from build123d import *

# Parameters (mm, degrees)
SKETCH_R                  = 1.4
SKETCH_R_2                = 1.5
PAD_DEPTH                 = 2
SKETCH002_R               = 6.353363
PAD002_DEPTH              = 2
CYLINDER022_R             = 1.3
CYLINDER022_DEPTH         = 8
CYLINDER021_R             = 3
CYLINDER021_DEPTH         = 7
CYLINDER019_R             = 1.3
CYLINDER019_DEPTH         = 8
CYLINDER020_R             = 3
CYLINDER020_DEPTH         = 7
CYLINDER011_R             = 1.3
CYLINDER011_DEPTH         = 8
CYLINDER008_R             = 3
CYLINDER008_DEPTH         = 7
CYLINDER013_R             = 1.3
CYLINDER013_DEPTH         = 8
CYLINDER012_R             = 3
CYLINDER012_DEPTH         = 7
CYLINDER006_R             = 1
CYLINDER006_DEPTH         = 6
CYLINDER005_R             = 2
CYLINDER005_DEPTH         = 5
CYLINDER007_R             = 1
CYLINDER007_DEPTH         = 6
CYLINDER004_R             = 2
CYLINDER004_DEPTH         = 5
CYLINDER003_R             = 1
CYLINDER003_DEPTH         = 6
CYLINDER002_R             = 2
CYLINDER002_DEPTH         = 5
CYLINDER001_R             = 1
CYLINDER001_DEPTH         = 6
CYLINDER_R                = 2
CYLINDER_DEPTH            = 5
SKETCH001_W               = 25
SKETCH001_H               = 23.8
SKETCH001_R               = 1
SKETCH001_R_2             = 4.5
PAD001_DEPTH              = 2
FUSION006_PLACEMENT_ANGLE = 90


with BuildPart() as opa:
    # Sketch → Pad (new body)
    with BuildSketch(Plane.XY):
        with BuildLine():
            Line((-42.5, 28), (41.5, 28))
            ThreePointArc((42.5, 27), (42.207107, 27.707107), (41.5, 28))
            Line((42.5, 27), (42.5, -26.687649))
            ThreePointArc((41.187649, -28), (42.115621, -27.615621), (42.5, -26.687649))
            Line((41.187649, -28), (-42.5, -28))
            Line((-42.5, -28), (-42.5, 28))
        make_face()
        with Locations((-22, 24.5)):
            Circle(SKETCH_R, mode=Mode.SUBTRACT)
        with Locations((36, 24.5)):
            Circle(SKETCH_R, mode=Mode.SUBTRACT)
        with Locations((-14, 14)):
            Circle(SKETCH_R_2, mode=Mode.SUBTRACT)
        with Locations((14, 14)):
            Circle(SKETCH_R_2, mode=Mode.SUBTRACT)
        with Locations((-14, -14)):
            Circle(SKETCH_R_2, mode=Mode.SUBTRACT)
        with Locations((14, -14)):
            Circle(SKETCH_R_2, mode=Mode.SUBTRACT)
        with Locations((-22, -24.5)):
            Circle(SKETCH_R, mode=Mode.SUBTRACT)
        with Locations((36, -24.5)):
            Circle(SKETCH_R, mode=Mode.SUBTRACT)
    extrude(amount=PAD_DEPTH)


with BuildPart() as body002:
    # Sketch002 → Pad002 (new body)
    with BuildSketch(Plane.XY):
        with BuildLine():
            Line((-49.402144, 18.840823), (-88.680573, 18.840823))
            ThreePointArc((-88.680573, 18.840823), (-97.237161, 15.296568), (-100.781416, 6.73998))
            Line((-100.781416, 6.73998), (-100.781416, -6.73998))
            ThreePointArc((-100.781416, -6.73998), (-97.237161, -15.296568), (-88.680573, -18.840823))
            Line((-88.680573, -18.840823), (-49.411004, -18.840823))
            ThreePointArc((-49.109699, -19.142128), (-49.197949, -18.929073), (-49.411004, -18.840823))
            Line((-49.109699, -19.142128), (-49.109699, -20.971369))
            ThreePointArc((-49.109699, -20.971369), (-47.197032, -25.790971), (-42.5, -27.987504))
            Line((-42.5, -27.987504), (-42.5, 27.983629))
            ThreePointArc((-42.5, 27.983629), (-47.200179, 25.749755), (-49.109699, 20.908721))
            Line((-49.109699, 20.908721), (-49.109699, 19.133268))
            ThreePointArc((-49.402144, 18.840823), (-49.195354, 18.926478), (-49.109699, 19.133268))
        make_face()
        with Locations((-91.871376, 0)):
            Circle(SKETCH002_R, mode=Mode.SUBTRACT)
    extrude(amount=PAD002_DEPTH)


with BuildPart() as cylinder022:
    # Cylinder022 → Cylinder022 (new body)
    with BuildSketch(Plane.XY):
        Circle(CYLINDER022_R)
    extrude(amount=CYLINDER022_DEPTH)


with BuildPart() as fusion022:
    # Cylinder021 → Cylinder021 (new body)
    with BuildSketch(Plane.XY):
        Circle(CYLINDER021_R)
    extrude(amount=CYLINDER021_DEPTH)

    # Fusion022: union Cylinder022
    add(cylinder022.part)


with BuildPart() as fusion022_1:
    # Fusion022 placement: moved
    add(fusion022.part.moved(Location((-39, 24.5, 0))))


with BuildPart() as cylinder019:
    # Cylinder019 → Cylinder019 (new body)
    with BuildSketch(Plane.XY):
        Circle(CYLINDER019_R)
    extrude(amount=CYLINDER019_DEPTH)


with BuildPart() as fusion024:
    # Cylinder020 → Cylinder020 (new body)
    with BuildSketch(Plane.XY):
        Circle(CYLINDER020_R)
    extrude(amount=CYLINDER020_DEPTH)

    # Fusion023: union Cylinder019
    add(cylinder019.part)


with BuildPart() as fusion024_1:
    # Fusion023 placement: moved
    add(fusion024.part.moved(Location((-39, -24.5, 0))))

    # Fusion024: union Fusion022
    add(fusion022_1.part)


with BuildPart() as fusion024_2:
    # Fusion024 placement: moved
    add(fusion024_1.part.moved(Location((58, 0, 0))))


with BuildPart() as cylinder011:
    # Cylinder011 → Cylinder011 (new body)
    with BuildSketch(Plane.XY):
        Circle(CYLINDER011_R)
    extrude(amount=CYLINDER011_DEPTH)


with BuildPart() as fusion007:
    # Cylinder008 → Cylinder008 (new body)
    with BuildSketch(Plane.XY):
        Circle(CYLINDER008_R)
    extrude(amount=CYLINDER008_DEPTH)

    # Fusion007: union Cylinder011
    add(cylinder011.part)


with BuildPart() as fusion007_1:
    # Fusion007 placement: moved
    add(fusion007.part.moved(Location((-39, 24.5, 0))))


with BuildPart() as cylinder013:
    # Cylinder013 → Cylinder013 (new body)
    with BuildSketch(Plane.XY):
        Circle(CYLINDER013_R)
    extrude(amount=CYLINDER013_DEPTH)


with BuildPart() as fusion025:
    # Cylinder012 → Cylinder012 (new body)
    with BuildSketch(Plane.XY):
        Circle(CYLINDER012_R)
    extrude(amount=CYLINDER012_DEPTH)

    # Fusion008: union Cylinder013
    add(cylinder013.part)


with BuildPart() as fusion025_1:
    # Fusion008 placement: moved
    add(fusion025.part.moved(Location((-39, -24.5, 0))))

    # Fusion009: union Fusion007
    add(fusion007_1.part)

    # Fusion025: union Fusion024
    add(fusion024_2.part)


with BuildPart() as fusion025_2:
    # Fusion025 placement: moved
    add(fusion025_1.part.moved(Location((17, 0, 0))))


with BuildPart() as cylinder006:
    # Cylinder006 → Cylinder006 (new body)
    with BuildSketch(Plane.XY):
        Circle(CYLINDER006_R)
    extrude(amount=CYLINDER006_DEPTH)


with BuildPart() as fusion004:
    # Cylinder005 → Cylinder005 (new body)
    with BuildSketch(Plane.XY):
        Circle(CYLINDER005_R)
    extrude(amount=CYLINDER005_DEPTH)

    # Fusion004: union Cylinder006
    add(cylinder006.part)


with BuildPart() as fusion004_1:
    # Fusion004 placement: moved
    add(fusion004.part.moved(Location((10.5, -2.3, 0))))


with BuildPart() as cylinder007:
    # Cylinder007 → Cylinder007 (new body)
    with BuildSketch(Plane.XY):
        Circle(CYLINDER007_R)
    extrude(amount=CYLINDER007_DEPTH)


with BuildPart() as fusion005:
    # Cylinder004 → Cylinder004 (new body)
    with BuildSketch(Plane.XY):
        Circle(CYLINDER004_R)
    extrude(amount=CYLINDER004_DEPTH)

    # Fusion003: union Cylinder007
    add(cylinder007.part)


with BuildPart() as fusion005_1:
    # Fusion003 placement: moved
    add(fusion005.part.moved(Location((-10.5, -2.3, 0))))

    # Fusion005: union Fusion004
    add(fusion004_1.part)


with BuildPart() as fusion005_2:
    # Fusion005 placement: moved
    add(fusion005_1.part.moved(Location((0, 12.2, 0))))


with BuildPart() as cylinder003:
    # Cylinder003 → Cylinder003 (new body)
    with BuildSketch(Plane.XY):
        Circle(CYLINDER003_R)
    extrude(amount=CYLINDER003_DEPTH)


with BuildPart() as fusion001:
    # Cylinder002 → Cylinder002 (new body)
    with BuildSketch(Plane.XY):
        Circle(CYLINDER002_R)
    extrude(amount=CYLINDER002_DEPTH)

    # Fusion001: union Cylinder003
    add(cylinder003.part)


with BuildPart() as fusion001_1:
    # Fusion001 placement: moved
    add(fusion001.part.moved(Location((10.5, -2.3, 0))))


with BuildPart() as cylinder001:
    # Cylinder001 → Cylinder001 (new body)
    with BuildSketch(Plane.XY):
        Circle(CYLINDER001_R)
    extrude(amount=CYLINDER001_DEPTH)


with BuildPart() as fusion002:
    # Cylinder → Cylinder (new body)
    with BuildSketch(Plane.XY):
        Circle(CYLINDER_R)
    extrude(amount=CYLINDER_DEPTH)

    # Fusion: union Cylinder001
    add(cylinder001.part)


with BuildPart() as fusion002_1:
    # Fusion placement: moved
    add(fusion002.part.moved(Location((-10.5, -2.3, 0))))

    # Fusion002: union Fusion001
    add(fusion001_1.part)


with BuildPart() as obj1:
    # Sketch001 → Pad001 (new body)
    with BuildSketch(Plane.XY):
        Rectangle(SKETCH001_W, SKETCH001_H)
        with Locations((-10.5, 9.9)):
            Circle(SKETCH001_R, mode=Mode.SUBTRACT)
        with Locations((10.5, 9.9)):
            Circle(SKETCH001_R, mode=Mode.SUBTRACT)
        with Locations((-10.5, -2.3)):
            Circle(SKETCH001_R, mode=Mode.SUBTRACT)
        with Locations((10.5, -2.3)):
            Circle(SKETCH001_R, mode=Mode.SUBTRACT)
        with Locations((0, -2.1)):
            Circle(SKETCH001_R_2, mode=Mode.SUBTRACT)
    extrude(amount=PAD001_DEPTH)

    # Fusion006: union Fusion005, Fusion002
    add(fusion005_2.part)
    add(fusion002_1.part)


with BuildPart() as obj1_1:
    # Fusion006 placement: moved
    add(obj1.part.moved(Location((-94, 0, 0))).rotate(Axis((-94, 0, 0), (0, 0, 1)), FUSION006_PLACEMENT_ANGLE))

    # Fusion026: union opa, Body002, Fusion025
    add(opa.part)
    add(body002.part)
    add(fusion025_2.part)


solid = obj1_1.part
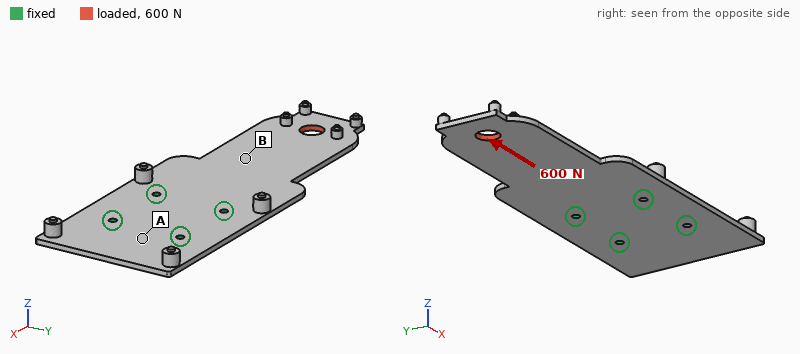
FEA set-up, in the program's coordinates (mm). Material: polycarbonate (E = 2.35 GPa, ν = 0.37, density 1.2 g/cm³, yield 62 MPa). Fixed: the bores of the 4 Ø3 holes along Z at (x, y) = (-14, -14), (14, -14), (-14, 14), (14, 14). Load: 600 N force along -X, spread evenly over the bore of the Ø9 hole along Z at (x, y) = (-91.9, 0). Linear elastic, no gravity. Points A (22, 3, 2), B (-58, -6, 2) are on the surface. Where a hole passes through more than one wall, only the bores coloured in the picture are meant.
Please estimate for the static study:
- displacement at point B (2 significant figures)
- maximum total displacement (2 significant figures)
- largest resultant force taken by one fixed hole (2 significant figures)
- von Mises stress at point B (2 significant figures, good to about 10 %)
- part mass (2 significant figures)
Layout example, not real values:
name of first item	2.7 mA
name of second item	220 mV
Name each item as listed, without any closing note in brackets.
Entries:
displacement at point B	0.14 mm
maximum total displacement	0.34 mm
largest resultant force taken by one fixed hole	240 N
von Mises stress at point B	7.4 MPa
part mass	18 g
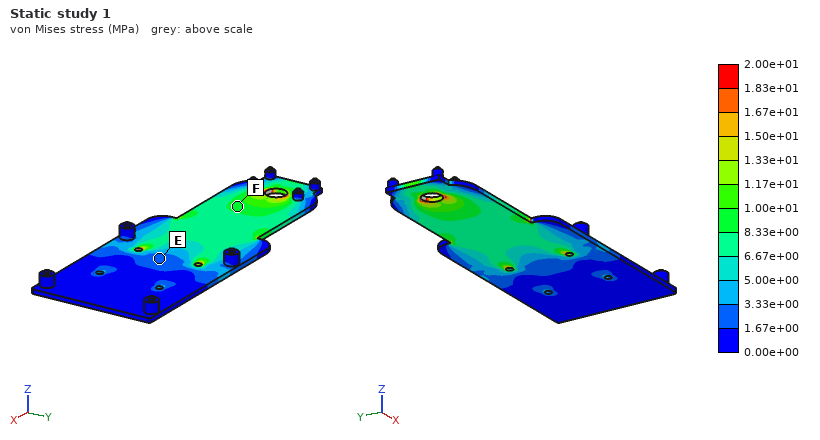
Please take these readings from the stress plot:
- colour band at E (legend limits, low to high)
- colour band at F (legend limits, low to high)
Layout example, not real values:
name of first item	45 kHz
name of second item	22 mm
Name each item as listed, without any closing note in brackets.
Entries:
colour band at E	1.67e+00 to 3.33e+00 MPa
colour band at F	8.33e+00 to 1.00e+01 MPa
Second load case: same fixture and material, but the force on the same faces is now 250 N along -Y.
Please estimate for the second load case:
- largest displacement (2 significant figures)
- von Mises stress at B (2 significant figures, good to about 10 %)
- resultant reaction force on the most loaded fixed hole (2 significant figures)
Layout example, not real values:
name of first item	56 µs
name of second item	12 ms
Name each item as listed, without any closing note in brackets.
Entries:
largest displacement	1.8 mm
von Mises stress at B	8.5 MPa
resultant reaction force on the most loaded fixed hole	450 N
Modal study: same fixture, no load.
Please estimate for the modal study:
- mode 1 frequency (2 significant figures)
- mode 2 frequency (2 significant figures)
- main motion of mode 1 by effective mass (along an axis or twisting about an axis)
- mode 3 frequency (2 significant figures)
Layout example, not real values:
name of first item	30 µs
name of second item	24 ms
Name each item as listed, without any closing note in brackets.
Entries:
mode 1 frequency	66 Hz
mode 2 frequency	310 Hz
main motion of mode 1 by effective mass	along Z
mode 3 frequency	350 Hz
